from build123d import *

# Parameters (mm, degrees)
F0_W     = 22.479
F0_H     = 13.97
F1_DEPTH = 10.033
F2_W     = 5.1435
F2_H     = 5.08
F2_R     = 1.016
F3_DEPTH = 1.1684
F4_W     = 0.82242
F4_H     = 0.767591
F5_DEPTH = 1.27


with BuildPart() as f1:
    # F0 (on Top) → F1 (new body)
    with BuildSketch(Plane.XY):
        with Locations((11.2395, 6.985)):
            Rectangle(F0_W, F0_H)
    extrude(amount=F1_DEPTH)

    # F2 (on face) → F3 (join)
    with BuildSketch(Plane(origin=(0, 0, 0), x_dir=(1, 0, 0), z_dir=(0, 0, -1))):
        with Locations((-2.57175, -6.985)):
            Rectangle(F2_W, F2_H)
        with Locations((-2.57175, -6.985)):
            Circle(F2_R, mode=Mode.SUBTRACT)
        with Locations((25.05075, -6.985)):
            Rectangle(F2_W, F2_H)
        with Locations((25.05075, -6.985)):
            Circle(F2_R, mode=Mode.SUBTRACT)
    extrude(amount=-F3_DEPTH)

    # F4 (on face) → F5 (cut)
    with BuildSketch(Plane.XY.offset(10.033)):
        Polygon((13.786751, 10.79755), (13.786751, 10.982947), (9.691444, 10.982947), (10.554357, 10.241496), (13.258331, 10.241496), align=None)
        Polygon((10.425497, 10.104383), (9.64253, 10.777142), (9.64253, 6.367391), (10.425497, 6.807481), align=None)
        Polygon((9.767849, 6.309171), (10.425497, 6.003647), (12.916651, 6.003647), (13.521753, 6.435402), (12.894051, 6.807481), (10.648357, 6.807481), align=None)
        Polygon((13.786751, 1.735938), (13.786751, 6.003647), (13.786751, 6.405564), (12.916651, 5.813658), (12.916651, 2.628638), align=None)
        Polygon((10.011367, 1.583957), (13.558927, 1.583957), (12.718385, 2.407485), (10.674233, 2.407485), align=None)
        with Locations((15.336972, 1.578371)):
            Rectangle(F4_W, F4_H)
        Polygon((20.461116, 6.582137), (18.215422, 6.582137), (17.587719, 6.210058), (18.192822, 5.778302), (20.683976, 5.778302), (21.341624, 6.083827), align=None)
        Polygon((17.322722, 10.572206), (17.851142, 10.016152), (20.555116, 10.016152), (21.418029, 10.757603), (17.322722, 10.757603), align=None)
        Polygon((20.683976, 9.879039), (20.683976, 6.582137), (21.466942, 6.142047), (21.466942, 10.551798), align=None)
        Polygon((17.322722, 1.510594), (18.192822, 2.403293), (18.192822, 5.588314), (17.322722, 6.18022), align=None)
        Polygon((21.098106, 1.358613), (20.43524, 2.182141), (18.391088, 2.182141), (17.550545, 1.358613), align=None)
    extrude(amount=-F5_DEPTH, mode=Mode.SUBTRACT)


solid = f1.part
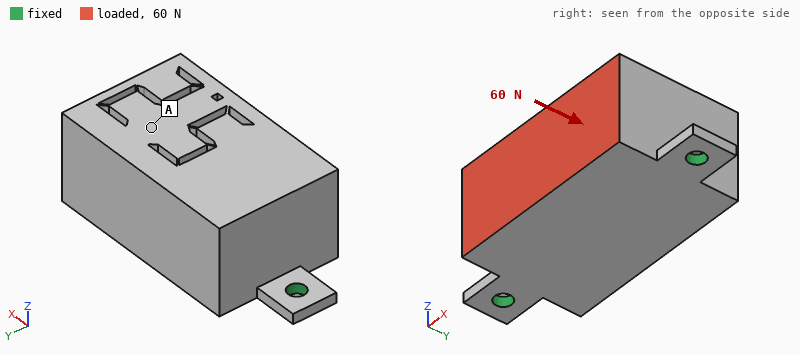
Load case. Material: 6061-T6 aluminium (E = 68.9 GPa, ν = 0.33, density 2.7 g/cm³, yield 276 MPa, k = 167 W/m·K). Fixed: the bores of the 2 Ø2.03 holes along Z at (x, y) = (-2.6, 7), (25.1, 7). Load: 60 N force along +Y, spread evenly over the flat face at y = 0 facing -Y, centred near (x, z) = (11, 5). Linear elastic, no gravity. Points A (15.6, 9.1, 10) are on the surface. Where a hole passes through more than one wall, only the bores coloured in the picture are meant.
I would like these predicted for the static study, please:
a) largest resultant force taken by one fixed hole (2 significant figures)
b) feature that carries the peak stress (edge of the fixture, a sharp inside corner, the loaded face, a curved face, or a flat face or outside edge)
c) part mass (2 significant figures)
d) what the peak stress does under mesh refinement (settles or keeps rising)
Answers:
30 N
edge of the fixture
8.6 g
keeps rising
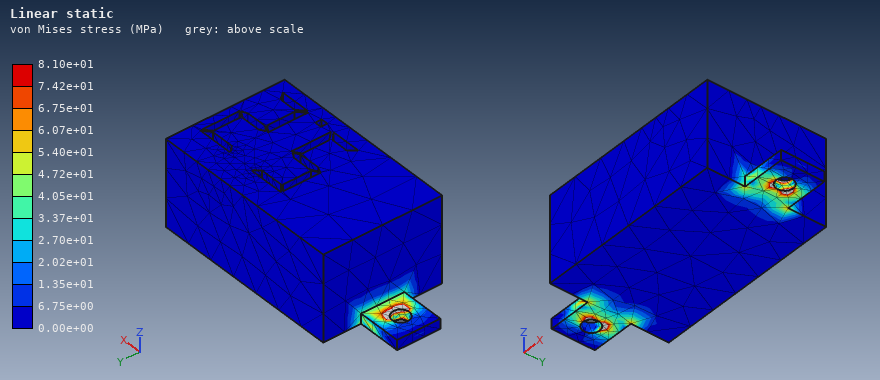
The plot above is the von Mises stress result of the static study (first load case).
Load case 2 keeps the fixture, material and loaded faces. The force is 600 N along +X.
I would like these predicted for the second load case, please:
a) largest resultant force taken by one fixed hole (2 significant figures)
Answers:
360 N
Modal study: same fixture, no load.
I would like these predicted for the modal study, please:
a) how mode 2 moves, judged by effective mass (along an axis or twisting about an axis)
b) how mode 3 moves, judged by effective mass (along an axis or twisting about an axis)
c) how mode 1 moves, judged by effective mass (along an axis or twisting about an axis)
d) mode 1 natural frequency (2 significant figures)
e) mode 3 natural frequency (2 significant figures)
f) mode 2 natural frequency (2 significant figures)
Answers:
along Z
along X
along Y
2500 Hz
16 kHz
11 kHz
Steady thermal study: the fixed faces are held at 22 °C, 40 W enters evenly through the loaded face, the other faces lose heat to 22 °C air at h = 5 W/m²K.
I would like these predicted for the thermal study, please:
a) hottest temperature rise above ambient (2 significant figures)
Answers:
75 K
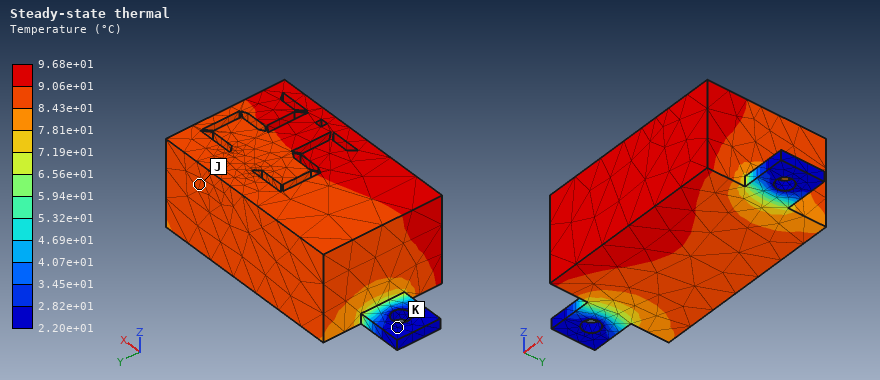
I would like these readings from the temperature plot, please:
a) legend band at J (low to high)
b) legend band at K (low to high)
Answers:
8.43e+01 to 9.06e+01 °C
2.20e+01 to 2.82e+01 °C
